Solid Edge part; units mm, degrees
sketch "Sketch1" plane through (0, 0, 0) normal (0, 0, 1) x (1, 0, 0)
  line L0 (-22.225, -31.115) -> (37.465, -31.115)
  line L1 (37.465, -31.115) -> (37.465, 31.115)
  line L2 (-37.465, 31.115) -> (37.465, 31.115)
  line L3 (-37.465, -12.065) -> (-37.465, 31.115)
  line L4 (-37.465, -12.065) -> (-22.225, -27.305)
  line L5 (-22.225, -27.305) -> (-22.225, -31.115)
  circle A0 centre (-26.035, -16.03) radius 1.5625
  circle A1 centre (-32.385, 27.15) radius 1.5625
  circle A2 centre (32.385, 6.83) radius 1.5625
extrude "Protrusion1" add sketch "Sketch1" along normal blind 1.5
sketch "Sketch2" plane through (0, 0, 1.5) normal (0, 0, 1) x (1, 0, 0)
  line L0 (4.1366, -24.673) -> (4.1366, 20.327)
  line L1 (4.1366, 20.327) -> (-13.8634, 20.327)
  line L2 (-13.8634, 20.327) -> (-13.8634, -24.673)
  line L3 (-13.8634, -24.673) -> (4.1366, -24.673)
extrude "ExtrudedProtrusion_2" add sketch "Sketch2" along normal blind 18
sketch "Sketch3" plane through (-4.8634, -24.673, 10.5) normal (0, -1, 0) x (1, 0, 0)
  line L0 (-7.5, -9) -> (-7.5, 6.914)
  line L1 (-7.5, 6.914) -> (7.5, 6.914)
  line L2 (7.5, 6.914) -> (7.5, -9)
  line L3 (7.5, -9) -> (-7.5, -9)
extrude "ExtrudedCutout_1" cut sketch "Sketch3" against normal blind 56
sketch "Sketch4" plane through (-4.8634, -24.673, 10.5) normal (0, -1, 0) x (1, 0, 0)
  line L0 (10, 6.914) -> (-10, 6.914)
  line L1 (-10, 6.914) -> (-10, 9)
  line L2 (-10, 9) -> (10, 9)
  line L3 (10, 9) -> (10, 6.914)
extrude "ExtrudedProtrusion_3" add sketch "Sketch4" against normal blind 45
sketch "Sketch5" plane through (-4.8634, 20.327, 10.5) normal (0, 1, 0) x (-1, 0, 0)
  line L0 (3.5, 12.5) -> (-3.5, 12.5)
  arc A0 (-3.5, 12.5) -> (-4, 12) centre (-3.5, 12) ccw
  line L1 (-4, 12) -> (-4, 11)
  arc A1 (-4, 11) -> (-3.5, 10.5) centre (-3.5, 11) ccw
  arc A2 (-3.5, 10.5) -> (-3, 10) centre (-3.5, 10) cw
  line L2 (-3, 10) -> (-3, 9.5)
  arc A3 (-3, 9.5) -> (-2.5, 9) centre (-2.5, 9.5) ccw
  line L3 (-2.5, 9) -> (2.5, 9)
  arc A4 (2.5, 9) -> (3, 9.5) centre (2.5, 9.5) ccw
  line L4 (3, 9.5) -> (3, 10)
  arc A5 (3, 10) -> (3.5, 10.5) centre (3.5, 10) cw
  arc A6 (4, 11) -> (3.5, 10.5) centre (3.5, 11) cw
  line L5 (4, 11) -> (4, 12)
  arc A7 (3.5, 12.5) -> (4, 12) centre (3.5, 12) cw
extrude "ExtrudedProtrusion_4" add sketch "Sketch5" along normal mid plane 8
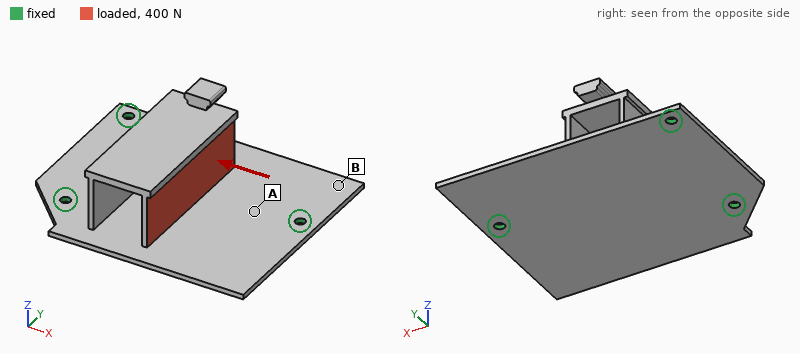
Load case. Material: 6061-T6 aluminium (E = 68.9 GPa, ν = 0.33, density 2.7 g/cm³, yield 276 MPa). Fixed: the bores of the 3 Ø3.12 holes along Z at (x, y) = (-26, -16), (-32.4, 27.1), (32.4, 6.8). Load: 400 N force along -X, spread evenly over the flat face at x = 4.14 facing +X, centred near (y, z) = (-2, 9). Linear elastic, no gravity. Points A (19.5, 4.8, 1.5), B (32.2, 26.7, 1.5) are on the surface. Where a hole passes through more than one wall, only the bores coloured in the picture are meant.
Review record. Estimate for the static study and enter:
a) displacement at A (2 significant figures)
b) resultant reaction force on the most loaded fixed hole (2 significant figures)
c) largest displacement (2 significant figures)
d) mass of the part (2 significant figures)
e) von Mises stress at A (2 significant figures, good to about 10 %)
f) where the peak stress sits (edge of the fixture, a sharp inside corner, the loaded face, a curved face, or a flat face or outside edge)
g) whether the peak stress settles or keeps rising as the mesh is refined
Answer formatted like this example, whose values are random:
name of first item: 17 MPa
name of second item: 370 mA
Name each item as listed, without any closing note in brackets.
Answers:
displacement at A: 0.068 mm
resultant reaction force on the most loaded fixed hole: 170 N
largest displacement: 0.20 mm
mass of the part: 29 g
von Mises stress at A: 23 MPa
where the peak stress sits: edge of the fixture
whether the peak stress settles or keeps rising as the mesh is refined: keeps rising
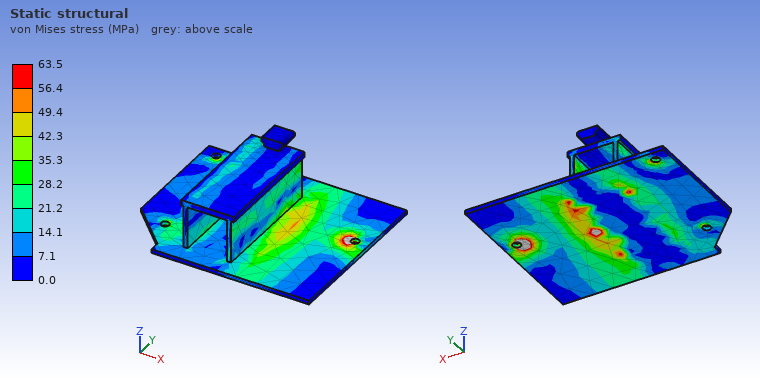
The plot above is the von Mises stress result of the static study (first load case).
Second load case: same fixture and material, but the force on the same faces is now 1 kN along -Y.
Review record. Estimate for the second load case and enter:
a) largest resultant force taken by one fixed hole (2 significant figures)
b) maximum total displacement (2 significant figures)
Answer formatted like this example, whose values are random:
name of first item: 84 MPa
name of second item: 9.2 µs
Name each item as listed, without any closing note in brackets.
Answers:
largest resultant force taken by one fixed hole: 430 N
maximum total displacement: 0.56 mm
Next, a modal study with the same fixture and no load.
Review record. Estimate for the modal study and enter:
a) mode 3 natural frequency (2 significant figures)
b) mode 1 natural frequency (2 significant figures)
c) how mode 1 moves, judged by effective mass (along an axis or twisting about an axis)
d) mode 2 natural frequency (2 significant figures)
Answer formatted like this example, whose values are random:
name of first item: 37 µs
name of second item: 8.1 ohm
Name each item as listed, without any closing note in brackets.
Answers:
mode 3 natural frequency: 2100 Hz
mode 1 natural frequency: 1100 Hz
how mode 1 moves, judged by effective mass: along Z
mode 2 natural frequency: 1300 Hz
